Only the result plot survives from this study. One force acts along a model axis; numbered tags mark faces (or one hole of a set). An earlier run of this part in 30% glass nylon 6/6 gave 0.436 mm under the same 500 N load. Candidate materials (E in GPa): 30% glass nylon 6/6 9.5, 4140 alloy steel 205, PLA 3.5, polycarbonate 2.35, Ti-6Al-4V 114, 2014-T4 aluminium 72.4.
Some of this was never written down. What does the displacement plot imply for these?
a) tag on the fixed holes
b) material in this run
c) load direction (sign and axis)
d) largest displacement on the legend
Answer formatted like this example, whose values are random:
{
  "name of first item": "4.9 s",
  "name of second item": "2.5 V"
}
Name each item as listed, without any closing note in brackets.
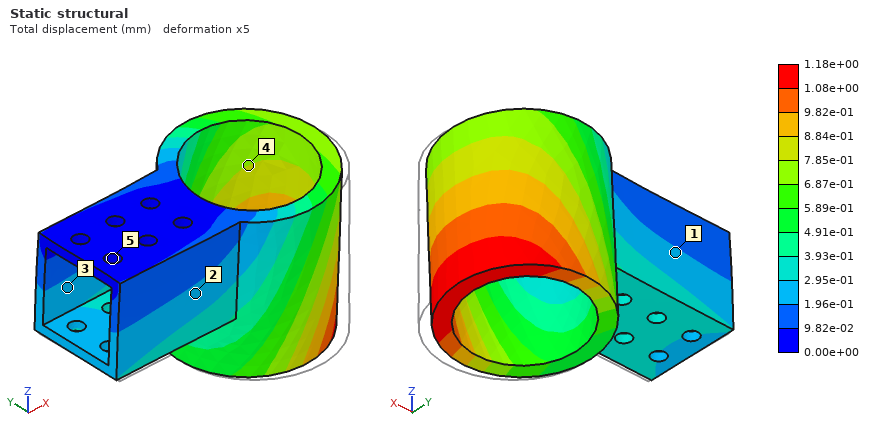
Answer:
{
  "tag on the fixed holes": "5",
  "material in this run": "PLA",
  "load direction": "+Y",
  "largest displacement on the legend": "1.18e+00 mm"
}
